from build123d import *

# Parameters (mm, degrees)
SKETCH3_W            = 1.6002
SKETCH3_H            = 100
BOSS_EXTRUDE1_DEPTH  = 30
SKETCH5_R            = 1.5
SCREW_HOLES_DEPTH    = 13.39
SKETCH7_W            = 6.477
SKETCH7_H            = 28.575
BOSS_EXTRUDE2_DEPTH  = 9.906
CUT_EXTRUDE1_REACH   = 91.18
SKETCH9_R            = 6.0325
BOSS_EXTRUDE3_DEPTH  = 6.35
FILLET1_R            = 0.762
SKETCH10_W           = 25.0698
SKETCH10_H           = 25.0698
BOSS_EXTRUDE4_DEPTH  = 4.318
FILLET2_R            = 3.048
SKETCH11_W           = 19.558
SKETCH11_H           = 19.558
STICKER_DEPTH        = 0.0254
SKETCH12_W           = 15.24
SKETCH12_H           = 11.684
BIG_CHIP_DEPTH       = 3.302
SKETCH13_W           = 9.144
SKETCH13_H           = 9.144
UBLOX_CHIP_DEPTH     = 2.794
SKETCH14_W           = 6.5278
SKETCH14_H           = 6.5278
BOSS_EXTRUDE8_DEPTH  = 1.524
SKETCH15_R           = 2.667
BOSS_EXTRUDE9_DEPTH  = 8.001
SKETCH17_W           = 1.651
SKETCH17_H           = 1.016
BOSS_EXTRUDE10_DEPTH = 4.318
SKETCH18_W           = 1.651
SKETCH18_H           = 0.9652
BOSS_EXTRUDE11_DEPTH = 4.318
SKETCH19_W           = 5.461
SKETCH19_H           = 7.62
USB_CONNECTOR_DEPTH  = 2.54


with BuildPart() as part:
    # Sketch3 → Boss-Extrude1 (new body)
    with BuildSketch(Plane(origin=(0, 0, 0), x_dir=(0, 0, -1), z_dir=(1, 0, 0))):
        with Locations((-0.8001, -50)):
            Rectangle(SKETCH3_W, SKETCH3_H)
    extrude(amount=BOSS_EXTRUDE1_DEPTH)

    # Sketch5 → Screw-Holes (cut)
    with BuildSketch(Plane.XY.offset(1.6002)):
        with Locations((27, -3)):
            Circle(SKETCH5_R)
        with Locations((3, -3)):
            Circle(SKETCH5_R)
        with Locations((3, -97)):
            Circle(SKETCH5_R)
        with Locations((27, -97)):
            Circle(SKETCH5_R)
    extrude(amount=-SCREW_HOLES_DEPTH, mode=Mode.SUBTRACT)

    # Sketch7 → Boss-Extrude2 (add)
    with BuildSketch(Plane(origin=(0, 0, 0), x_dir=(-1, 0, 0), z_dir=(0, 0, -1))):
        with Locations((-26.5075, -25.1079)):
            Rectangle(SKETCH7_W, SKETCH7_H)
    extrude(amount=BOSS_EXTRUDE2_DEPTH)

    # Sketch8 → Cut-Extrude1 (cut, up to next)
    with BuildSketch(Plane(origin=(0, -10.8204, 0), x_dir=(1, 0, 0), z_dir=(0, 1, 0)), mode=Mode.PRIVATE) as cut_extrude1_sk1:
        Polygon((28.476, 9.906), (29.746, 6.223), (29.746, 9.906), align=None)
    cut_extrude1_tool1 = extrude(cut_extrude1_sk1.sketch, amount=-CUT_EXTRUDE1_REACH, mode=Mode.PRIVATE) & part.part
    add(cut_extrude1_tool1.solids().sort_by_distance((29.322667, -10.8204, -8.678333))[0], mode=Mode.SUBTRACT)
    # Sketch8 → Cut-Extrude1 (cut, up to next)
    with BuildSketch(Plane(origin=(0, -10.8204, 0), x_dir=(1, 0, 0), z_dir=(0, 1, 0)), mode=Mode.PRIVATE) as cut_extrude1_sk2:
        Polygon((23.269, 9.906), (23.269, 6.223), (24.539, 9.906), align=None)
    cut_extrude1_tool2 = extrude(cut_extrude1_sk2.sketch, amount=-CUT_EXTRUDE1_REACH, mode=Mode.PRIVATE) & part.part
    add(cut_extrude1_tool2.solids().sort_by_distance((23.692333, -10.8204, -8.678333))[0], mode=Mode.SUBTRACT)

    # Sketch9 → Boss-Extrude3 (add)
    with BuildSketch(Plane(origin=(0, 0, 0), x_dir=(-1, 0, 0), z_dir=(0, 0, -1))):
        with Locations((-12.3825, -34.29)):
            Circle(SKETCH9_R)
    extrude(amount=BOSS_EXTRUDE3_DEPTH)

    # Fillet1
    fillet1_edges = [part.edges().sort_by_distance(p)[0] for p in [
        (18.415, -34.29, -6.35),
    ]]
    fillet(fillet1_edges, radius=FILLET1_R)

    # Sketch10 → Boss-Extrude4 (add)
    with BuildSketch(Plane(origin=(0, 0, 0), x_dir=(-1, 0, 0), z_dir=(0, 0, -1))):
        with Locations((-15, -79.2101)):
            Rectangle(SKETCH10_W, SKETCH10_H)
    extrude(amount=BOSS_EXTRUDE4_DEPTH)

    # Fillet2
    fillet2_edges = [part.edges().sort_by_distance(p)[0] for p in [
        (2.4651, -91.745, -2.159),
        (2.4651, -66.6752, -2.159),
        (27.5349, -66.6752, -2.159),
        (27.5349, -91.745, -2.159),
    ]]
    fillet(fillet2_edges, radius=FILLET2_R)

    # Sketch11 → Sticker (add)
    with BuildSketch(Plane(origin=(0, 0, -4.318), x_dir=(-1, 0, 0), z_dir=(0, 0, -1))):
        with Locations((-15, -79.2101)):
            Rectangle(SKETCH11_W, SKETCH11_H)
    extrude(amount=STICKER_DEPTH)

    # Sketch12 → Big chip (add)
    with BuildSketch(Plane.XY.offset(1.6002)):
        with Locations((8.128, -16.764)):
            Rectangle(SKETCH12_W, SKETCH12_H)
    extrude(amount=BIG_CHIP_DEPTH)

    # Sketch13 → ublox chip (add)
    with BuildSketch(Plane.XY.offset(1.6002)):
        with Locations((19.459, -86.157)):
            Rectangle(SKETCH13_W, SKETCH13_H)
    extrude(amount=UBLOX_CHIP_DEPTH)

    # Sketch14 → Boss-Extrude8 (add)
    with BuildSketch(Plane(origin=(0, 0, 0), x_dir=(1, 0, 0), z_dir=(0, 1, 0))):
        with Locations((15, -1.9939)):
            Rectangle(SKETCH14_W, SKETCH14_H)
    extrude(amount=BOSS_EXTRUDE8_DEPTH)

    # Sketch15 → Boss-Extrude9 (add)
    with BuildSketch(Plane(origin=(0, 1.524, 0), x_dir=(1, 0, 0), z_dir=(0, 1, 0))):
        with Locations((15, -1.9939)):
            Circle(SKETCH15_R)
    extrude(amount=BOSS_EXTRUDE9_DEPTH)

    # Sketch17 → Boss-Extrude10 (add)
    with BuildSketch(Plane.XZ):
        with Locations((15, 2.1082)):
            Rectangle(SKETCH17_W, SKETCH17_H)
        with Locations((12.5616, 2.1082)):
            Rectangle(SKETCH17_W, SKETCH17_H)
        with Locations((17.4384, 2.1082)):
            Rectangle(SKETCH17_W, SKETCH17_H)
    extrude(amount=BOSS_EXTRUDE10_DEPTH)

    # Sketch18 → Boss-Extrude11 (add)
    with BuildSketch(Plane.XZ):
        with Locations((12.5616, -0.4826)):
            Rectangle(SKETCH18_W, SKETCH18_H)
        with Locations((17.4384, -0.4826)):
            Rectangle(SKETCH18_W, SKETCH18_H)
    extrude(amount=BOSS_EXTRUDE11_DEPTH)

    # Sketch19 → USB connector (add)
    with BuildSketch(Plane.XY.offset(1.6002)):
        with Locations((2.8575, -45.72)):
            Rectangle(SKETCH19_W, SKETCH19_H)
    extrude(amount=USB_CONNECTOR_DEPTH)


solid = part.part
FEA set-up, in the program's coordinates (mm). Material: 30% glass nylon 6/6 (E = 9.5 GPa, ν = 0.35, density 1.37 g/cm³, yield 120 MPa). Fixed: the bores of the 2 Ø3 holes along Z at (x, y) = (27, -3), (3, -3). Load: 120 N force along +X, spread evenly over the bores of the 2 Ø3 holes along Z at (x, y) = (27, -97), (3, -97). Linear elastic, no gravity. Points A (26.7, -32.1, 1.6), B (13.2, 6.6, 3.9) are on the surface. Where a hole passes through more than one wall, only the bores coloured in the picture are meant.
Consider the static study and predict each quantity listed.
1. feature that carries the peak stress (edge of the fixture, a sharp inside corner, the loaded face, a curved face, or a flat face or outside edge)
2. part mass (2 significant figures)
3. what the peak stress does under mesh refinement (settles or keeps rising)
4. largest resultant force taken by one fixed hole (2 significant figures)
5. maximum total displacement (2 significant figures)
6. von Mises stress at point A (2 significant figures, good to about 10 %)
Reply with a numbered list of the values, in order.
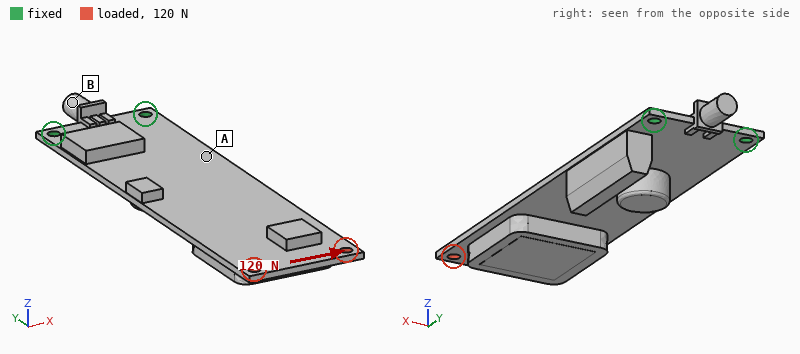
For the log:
1. edge of the fixture
2. 15 g
3. keeps rising
4. 470 N
5. 1.3 mm
6. 16 MPa
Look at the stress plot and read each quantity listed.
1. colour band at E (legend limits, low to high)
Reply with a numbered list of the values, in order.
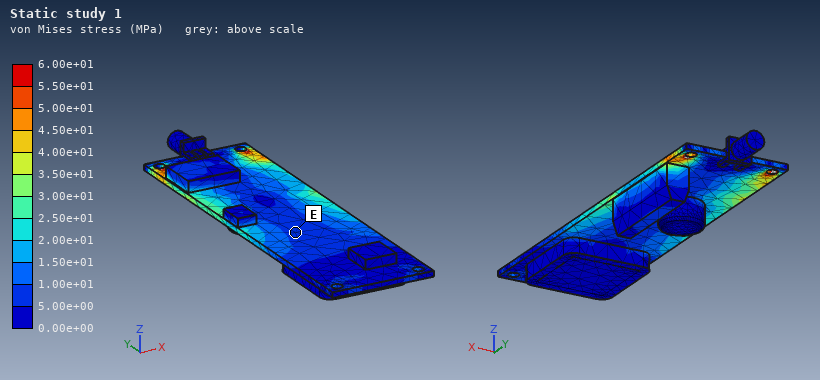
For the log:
1. 5.00e+00 to 1.00e+01 MPa
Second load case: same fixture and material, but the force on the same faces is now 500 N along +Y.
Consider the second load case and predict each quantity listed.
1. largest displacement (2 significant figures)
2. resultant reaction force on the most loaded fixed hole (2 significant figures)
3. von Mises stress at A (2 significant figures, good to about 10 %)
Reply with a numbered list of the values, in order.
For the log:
1. 0.25 mm
2. 260 N
3. 6.9 MPa
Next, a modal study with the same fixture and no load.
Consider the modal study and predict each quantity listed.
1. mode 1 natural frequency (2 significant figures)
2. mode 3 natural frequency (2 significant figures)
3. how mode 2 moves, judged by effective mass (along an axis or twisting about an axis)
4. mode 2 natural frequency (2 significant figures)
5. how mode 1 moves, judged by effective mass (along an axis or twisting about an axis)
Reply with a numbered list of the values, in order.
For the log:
1. 67 Hz
2. 560 Hz
3. along Z
4. 400 Hz
5. along Z
